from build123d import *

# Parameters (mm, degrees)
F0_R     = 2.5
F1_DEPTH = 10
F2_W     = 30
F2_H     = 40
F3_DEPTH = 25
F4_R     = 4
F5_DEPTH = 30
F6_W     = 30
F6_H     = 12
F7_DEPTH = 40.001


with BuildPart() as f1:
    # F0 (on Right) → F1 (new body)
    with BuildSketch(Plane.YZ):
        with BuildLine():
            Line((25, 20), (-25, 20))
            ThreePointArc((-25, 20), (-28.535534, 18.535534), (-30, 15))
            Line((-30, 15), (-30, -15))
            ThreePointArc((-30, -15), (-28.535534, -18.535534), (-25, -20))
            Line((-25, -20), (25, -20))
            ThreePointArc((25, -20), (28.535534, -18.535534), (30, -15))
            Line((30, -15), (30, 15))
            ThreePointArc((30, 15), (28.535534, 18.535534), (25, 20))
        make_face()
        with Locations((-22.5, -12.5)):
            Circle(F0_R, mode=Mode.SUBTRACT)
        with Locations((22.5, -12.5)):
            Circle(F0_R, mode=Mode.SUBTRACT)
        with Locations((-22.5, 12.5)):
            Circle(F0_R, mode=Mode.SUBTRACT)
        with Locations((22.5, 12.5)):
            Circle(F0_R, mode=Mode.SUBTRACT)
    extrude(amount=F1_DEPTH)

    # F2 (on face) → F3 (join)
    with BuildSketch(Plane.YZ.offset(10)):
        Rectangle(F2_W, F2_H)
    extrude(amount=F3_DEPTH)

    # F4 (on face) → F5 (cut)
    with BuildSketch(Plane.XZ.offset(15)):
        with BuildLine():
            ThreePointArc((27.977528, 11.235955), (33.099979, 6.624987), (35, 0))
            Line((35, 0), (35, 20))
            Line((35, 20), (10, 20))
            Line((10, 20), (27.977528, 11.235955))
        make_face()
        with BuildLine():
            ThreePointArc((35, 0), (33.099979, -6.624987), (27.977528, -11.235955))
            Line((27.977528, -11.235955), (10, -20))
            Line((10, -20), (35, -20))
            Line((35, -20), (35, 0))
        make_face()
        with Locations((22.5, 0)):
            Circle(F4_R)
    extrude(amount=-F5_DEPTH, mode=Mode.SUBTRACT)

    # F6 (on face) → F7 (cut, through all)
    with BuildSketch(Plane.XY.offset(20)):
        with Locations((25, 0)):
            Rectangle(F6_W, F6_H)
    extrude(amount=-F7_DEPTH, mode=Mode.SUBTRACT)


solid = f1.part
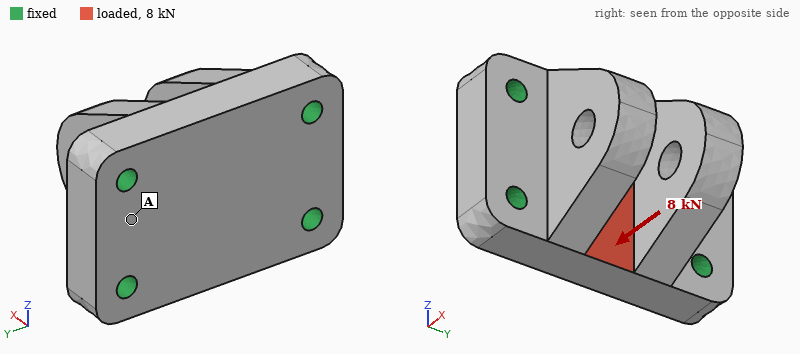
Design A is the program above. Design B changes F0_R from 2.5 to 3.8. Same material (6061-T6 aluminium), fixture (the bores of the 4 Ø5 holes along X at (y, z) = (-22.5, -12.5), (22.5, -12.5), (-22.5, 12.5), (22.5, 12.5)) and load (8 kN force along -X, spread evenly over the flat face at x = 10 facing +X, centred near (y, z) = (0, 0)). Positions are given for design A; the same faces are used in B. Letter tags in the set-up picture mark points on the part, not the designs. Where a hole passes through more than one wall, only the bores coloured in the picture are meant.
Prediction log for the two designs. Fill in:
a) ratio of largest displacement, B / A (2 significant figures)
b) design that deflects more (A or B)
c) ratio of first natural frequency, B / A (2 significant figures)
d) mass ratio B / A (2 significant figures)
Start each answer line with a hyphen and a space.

- 0.86
- A
- 1.0
- 0.97
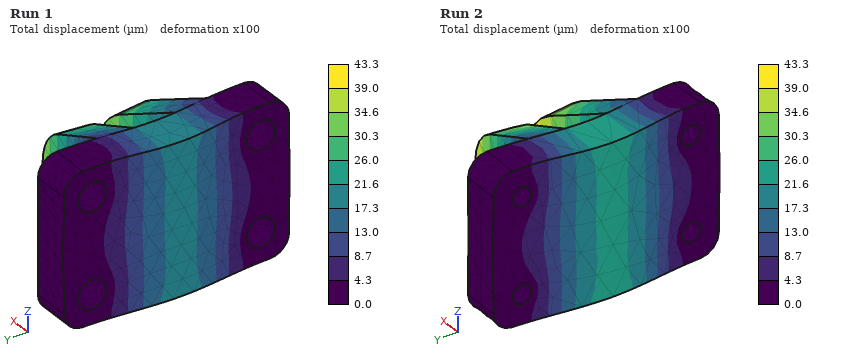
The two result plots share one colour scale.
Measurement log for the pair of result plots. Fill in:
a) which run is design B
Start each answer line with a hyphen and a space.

- Run 1
